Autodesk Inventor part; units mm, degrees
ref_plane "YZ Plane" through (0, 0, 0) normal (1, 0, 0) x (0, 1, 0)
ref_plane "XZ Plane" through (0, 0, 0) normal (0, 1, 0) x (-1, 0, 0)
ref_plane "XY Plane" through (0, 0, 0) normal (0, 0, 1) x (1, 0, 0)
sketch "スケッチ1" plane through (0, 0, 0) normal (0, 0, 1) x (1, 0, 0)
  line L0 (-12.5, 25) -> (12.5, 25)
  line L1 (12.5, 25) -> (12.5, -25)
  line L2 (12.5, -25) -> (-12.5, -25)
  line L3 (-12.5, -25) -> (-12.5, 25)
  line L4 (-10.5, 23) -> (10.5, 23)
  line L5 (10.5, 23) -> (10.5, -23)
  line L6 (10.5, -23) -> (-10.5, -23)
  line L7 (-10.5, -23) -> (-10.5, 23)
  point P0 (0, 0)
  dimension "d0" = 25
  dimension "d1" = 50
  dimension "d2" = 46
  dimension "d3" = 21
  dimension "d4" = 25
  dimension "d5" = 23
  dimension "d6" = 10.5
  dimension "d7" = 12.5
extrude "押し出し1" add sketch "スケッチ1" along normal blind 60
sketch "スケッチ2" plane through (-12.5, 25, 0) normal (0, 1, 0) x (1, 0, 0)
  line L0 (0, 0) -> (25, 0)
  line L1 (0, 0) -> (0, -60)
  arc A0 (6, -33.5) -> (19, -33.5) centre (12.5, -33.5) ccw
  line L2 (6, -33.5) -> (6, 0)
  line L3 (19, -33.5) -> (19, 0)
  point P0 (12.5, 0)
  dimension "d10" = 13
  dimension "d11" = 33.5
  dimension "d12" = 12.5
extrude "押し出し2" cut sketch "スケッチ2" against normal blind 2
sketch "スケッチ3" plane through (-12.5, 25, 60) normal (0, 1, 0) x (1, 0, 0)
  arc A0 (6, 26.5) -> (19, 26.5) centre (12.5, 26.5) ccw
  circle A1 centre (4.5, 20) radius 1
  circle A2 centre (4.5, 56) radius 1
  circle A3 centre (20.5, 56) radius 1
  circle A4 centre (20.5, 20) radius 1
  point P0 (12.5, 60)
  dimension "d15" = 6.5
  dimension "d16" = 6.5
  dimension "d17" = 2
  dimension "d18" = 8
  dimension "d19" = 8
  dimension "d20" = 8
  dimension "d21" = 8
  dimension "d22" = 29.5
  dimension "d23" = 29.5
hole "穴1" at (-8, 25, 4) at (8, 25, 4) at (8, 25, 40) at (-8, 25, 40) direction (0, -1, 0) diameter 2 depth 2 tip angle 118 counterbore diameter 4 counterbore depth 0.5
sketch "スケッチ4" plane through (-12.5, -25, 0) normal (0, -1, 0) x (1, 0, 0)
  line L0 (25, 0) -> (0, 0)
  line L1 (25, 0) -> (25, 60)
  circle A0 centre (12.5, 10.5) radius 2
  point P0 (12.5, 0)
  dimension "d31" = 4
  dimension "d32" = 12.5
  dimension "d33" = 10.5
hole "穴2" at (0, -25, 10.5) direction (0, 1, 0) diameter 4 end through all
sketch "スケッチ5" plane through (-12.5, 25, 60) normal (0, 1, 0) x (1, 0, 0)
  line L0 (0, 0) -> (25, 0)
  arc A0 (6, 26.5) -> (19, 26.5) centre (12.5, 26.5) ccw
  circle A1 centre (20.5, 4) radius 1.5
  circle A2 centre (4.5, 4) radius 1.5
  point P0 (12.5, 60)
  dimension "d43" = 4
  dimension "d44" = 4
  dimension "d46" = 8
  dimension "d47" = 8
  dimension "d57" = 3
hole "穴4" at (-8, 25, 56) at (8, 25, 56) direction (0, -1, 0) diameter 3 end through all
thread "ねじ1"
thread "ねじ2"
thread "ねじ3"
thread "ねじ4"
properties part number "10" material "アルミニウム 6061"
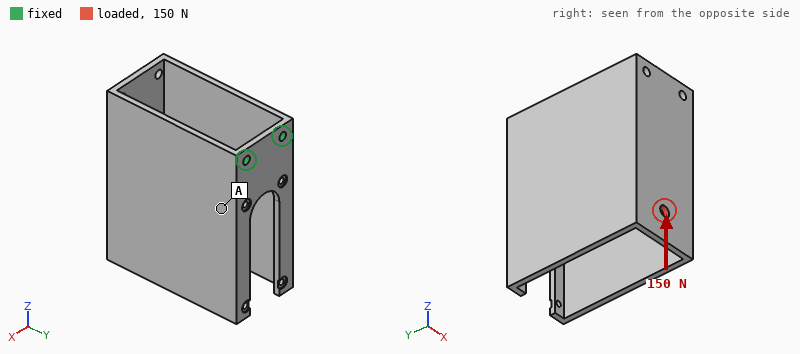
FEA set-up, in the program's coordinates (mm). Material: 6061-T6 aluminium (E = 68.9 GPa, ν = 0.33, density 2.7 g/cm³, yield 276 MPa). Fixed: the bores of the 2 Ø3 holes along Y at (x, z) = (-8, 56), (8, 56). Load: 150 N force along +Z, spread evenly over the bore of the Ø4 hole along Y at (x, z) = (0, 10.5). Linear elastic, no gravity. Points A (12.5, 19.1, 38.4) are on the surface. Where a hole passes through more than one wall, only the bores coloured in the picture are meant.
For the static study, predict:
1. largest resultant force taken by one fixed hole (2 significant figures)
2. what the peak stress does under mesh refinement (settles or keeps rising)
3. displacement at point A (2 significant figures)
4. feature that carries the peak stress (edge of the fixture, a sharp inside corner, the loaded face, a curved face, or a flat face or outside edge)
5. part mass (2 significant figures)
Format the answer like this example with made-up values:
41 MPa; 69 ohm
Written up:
75 N; keeps rising; 0.17 mm; edge of the fixture; 43 g
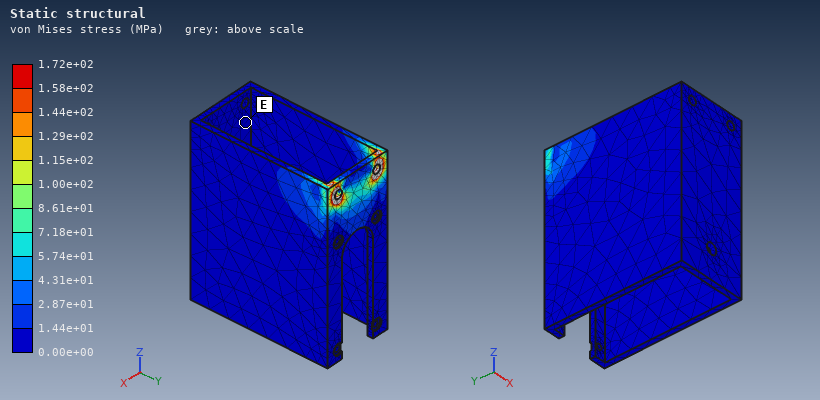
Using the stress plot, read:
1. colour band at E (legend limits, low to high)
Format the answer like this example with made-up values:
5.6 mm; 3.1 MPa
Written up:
0.00e+00 to 1.44e+01 MPa
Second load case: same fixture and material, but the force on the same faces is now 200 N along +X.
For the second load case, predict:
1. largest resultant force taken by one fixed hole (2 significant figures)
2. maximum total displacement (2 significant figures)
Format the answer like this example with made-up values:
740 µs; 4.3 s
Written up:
630 N; 0.83 mm
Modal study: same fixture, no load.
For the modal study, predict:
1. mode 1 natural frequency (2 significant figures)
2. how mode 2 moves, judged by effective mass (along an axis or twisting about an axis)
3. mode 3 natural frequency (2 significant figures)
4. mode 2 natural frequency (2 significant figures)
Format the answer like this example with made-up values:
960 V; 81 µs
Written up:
490 Hz; along X; 1100 Hz; 570 Hz
